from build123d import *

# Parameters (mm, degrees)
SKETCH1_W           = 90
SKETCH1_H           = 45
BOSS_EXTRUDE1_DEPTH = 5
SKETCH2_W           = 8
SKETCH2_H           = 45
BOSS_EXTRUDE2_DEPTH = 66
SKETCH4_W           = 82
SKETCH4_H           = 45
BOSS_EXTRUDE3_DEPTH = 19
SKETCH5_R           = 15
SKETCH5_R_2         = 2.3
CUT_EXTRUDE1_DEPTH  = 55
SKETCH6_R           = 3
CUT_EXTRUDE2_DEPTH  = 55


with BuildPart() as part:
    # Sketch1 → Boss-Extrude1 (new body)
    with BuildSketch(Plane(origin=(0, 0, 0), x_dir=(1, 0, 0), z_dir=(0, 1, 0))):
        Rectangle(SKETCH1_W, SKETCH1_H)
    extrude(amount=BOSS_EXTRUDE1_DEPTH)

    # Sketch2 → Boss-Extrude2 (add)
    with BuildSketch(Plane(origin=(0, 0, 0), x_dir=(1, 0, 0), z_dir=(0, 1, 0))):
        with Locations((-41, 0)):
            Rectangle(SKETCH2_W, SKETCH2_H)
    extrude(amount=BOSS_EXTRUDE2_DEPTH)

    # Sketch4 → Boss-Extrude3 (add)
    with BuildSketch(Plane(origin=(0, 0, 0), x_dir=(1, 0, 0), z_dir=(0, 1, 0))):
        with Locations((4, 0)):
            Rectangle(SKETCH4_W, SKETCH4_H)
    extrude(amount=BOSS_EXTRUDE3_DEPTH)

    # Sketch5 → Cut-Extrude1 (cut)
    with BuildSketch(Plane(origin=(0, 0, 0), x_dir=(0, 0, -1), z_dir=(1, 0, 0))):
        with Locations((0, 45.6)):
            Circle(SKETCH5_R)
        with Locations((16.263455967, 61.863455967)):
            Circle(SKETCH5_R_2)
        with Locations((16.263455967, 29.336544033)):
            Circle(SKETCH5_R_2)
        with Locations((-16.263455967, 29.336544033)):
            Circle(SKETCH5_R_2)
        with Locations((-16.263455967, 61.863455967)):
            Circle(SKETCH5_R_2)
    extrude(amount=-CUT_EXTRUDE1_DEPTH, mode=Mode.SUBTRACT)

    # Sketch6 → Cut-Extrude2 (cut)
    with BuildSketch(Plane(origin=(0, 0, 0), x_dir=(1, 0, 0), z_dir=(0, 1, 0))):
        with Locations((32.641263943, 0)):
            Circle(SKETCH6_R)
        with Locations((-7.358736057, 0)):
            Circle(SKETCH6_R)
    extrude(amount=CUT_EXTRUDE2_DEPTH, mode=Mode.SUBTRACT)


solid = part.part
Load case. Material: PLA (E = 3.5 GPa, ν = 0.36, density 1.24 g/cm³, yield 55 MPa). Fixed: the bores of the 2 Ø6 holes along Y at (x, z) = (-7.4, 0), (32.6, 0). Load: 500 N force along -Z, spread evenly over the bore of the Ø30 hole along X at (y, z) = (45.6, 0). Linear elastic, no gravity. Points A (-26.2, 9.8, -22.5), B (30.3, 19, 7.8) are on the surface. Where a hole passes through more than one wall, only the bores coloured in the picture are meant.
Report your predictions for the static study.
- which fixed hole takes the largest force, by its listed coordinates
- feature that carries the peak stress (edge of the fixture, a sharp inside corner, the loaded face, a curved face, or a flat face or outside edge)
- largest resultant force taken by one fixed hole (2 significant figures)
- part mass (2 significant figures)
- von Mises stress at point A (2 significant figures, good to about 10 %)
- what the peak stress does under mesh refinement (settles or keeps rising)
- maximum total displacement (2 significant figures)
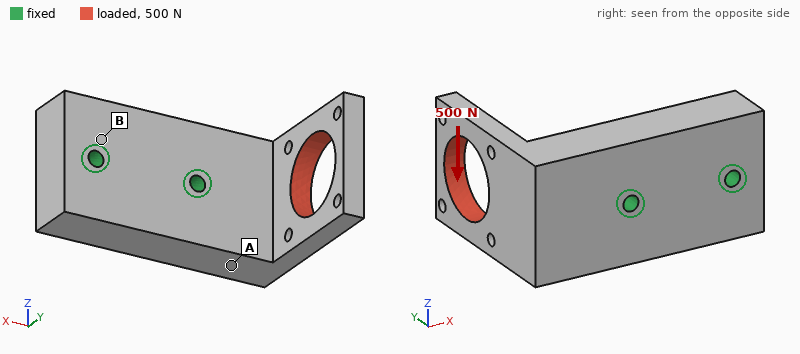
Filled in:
(-7.4, 0)
edge of the fixture
850 N
110 g
6.1 MPa
keeps rising
0.81 mm
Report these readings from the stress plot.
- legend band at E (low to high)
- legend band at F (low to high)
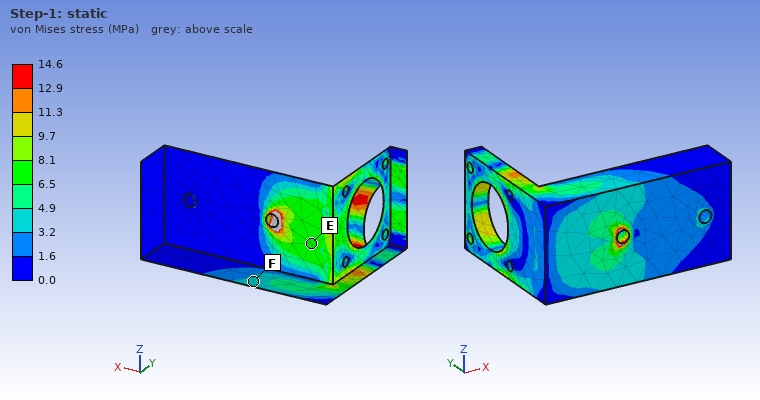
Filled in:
6.5 to 8.1 MPa
3.2 to 4.9 MPa
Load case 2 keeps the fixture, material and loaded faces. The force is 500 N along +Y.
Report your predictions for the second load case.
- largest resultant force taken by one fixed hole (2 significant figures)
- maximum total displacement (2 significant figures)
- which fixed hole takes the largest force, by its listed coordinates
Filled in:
660 N
0.32 mm
(-7.4, 0)
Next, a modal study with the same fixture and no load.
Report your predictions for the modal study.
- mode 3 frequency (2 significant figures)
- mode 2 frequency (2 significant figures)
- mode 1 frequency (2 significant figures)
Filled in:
1600 Hz
1300 Hz
750 Hz
